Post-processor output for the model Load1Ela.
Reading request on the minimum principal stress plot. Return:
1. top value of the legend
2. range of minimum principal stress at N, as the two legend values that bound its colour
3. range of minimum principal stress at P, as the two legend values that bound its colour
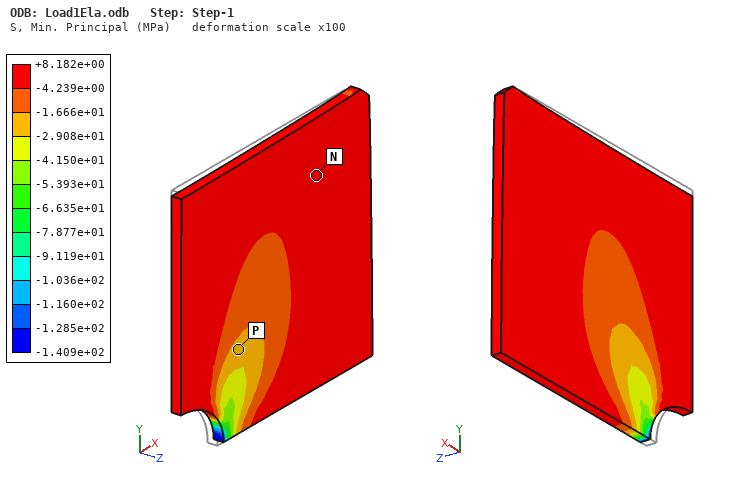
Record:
+8.182e+00 MPa
-4.239e+00 to +8.182e+00 MPa
-2.908e+01 to -1.666e+01 MPa
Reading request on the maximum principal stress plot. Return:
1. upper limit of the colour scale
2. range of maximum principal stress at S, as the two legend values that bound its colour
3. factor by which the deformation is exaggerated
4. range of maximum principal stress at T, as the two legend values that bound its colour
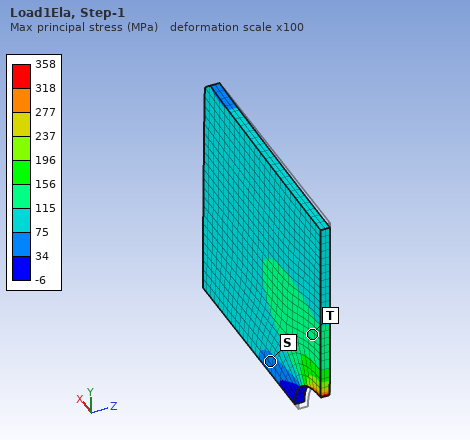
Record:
358 MPa
34 to 75 MPa
100
115 to 156 MPa
